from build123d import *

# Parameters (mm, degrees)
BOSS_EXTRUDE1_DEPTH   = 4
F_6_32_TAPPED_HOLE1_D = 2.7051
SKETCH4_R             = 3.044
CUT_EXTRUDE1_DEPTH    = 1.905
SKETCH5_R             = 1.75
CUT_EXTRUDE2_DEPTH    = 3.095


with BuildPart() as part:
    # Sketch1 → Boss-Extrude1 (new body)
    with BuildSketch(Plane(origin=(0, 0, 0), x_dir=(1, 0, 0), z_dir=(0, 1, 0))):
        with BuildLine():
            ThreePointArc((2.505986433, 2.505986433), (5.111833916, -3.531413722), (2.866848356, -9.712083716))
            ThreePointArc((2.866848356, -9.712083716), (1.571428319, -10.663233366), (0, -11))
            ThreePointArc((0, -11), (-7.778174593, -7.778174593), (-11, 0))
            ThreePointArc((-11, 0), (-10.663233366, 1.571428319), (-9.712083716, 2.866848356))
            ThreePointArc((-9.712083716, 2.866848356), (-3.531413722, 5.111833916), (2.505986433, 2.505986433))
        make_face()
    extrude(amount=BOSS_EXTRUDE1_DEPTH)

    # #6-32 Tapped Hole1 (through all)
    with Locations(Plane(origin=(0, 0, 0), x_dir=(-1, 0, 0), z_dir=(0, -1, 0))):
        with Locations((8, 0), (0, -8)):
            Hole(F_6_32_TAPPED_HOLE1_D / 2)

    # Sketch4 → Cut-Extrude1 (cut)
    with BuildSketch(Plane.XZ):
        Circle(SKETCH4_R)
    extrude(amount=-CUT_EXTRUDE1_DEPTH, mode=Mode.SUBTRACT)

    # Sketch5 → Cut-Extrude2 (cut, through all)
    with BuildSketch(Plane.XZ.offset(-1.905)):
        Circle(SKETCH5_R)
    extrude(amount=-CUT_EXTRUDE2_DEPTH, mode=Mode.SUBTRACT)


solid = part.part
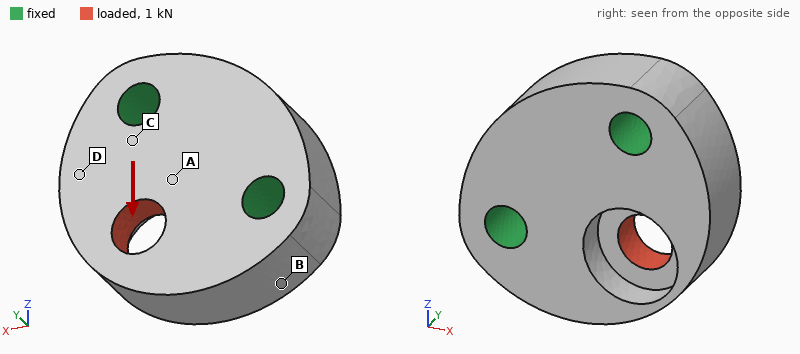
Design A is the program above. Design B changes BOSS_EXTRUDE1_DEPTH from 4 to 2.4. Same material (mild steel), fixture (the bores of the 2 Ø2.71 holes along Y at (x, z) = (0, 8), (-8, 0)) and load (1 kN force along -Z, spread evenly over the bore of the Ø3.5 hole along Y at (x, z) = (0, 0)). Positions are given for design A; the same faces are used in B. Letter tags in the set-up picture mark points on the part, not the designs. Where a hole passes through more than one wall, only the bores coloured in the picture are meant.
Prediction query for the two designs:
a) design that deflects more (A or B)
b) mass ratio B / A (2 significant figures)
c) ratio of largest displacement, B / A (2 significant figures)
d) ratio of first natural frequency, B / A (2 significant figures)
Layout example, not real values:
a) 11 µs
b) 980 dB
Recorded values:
a) B
b) 0.58
c) 3.2
d) 0.73
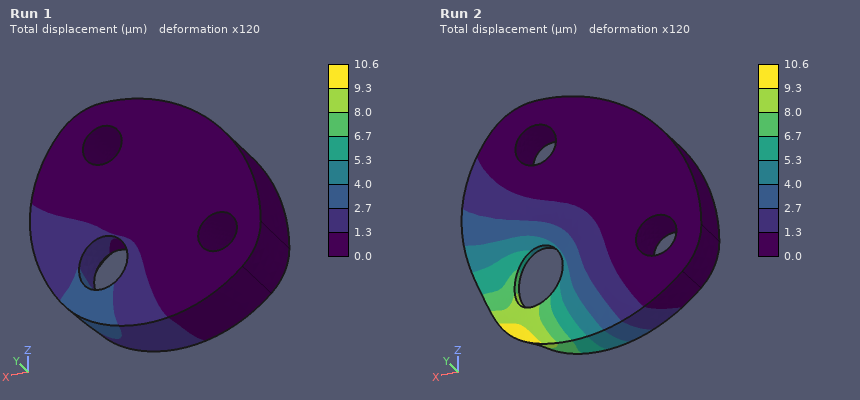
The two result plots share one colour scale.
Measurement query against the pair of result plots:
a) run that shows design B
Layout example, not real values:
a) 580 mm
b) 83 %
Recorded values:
a) Run 2
